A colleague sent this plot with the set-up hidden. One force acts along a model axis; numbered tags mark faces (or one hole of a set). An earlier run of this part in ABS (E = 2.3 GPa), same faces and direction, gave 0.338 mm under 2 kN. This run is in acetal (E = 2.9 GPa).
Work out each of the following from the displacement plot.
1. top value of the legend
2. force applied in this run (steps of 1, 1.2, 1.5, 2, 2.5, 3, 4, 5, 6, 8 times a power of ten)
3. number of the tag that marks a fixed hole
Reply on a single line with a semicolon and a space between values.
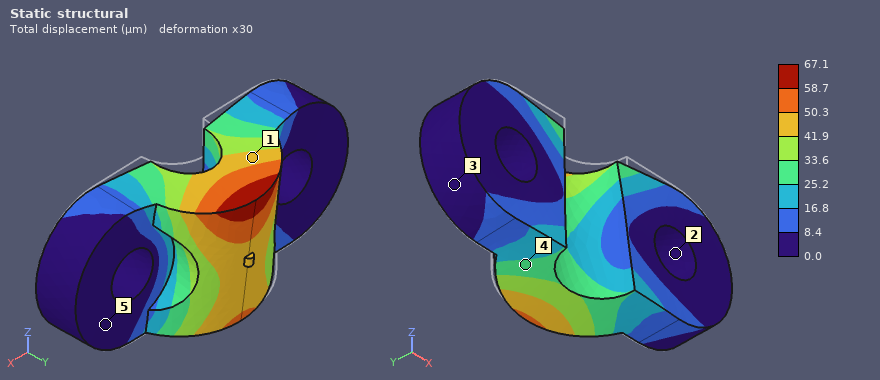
67.1 µm; 500 N; 2
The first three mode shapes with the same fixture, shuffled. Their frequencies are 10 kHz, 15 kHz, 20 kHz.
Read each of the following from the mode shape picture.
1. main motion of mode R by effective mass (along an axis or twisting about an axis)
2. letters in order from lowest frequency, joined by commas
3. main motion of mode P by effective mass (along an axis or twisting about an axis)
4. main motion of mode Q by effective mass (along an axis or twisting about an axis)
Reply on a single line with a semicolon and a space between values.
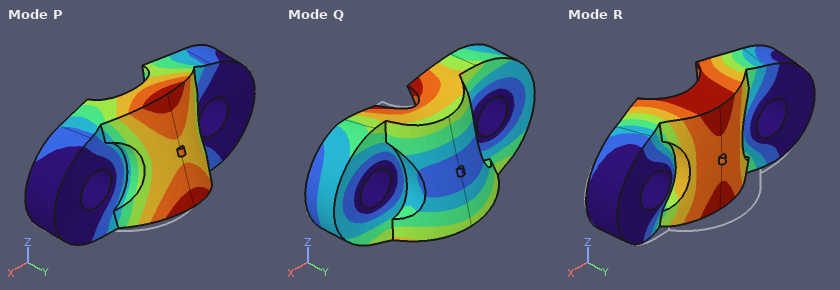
along Y; P, R, Q; along Z; along Z
